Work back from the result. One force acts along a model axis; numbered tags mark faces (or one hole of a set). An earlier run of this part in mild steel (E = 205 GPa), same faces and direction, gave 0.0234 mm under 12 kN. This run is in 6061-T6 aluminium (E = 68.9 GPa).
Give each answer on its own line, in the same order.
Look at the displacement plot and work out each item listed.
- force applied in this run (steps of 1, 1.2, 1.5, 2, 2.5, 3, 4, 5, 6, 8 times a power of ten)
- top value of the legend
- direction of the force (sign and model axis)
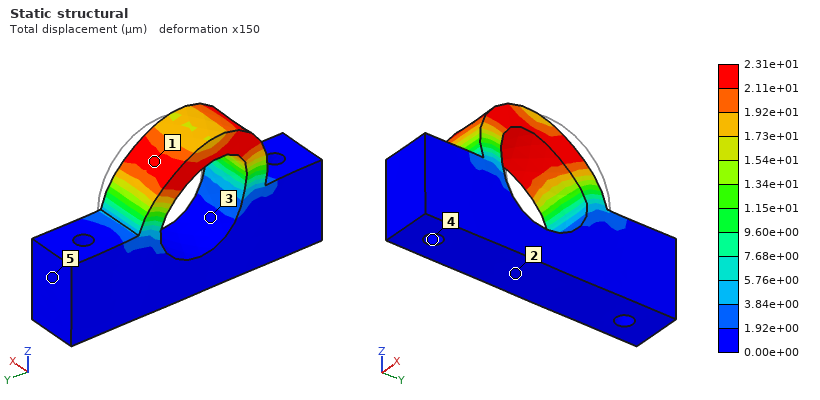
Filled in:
4 kN
2.31e+01 µm
-Y
